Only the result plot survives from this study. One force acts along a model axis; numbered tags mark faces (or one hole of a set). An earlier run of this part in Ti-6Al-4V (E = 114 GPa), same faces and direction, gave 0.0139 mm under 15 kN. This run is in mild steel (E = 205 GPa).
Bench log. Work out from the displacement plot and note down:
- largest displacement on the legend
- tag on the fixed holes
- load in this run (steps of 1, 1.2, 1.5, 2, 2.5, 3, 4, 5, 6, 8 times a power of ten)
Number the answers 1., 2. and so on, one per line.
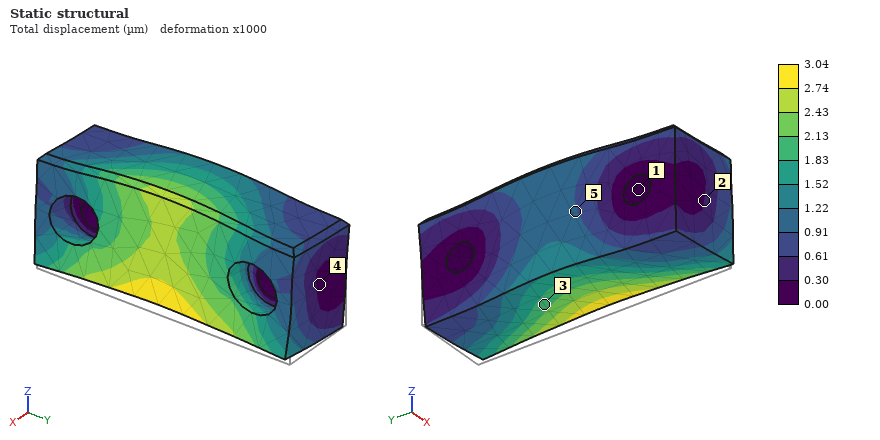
1. 3.04 µm
2. 1
3. 6 kN
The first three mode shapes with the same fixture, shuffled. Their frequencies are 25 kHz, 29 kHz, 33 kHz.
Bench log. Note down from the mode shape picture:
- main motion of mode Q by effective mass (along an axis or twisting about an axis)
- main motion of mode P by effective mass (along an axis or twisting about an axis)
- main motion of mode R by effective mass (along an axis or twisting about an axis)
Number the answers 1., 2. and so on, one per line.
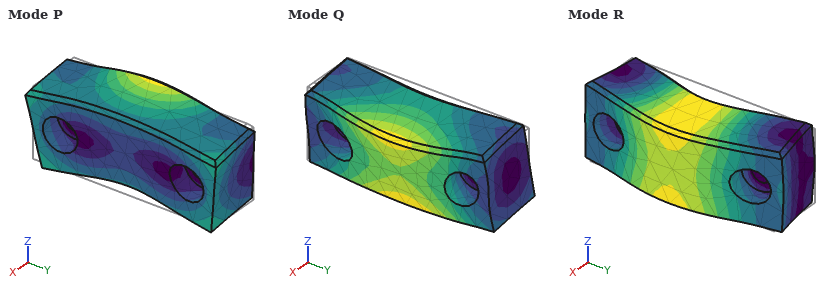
1. along Z
2. along Z
3. along X
